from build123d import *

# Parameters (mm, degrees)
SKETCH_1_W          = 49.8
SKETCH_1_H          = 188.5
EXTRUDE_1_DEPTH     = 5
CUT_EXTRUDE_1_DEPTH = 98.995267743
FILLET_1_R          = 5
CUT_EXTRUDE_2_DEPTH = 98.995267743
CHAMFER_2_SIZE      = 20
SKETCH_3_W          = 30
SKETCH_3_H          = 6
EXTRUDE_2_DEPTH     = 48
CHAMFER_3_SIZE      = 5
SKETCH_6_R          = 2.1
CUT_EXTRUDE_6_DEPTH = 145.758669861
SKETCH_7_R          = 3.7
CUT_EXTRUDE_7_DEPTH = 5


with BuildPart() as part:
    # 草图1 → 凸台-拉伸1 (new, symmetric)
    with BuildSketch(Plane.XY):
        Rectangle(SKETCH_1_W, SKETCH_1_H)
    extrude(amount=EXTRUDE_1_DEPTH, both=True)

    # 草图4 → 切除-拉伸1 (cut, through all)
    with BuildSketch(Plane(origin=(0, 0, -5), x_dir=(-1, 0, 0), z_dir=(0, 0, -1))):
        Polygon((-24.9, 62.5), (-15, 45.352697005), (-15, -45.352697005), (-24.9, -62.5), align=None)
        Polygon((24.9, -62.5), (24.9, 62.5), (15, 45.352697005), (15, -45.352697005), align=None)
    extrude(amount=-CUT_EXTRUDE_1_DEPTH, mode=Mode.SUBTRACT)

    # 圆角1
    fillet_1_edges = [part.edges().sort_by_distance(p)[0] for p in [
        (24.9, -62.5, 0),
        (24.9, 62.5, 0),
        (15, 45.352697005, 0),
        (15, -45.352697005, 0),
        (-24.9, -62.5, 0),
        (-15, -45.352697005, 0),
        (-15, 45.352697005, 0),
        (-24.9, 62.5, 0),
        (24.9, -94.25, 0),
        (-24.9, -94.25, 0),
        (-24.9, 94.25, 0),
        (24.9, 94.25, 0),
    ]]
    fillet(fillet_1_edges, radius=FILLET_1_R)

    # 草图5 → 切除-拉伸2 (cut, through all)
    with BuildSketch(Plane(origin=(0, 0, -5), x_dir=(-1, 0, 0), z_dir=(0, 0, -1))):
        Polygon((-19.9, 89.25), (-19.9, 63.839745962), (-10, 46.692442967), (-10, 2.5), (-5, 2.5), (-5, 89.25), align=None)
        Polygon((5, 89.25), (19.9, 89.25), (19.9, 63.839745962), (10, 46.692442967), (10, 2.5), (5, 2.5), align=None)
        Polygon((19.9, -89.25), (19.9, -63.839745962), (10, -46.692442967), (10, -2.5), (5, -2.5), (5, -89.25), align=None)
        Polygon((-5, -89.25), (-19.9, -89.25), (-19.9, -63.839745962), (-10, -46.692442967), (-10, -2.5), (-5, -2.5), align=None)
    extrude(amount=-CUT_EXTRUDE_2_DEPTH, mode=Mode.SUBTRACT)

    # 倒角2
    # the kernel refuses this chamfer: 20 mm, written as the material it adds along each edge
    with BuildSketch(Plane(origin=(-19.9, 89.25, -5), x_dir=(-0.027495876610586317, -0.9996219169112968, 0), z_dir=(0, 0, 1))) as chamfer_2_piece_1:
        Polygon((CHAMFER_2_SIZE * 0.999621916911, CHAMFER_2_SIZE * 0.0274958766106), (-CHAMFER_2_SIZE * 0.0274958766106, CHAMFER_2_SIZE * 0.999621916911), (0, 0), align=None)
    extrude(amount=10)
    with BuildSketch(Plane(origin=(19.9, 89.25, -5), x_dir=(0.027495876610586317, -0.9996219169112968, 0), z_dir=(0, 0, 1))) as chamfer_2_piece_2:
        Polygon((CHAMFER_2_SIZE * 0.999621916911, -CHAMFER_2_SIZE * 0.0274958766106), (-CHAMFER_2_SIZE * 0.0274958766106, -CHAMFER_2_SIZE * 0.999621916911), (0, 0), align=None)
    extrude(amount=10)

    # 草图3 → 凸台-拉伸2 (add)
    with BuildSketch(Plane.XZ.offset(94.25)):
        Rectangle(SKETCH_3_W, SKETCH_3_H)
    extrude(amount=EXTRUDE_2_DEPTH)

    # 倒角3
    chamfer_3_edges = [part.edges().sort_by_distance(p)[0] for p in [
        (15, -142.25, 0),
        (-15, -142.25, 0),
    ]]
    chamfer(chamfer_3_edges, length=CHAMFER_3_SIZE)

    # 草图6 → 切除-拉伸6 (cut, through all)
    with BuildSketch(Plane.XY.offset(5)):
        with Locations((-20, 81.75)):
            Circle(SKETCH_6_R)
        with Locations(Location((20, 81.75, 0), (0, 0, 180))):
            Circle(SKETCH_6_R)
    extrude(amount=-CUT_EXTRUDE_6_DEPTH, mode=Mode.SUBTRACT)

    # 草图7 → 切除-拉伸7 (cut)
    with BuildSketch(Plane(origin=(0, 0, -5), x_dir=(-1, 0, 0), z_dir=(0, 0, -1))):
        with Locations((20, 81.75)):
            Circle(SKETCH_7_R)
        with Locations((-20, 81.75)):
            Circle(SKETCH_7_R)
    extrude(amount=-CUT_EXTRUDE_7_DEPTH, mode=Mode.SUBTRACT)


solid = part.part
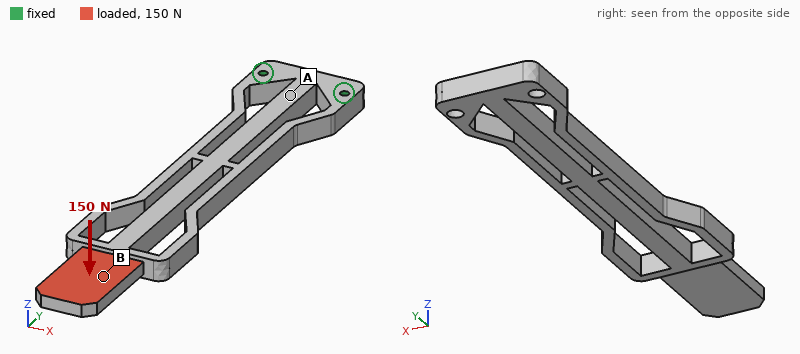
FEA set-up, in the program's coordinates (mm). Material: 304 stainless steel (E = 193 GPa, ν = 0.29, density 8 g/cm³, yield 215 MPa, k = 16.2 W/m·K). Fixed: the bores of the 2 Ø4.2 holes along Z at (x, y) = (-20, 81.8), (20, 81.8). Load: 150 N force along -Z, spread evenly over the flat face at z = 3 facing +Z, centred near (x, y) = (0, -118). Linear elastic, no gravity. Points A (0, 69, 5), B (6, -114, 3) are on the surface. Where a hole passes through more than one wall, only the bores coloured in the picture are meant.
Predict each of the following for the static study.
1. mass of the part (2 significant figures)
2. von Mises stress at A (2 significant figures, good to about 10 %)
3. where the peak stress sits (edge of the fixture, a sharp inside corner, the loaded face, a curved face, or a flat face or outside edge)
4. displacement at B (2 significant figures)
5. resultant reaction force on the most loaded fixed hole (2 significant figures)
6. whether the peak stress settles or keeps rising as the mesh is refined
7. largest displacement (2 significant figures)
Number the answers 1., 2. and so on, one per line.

1. 430 g
2. 72 MPa
3. edge of the fixture
4. 1.5 mm
5. 75 N
6. keeps rising
7. 1.8 mm
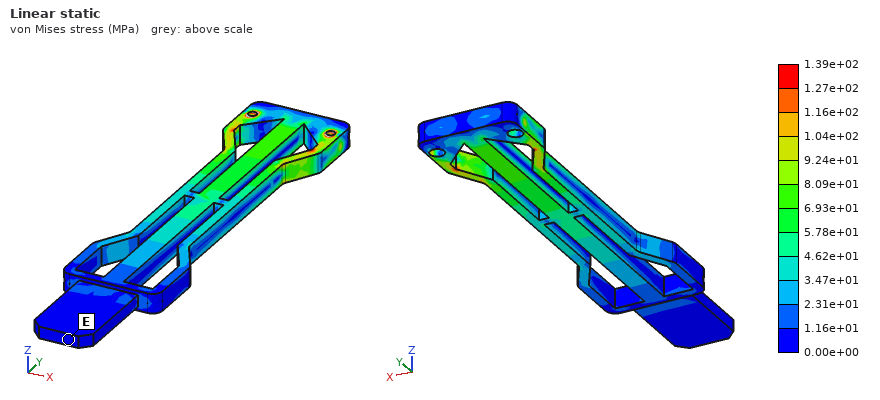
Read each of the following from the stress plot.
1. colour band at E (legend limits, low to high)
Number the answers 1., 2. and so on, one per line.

1. 0.00e+00 to 1.16e+01 MPa
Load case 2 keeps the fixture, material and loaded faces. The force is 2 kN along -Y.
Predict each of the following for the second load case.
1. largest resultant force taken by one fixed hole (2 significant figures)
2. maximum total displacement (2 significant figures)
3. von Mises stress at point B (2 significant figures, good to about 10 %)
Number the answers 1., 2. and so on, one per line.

1. 1.1 kN
2. 0.54 mm
3. 26 MPa
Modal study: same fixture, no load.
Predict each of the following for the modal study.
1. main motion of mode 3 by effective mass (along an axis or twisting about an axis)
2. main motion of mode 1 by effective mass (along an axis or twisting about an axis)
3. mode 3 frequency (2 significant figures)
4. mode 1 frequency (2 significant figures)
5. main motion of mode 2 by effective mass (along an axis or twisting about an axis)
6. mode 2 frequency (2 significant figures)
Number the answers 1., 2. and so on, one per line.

1. along Z
2. along Z
3. 870 Hz
4. 140 Hz
5. along X
6. 310 Hz
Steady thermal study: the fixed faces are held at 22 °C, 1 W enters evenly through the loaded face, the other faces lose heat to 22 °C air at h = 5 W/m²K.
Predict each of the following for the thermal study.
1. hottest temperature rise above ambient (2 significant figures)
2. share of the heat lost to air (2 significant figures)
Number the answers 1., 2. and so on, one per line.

1. 24 K
2. 86 %
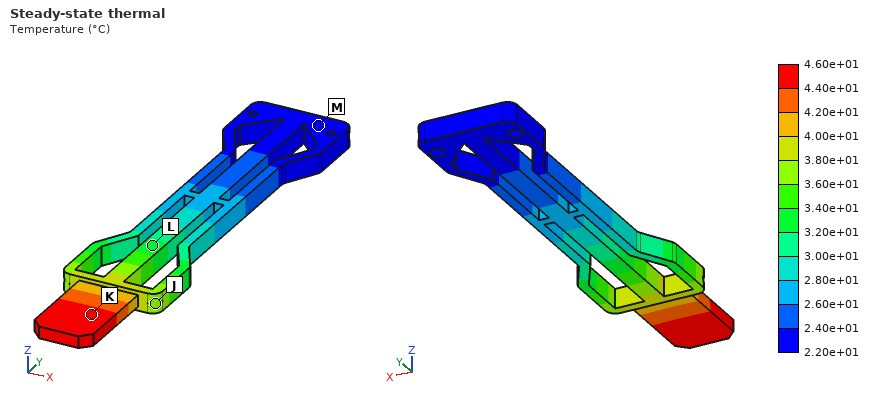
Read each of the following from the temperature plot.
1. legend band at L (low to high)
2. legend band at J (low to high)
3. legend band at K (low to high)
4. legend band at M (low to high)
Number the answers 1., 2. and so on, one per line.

1. 3.20e+01 to 3.40e+01 °C
2. 3.60e+01 to 3.80e+01 °C
3. 4.40e+01 to 4.60e+01 °C
4. 2.20e+01 to 2.40e+01 °C
